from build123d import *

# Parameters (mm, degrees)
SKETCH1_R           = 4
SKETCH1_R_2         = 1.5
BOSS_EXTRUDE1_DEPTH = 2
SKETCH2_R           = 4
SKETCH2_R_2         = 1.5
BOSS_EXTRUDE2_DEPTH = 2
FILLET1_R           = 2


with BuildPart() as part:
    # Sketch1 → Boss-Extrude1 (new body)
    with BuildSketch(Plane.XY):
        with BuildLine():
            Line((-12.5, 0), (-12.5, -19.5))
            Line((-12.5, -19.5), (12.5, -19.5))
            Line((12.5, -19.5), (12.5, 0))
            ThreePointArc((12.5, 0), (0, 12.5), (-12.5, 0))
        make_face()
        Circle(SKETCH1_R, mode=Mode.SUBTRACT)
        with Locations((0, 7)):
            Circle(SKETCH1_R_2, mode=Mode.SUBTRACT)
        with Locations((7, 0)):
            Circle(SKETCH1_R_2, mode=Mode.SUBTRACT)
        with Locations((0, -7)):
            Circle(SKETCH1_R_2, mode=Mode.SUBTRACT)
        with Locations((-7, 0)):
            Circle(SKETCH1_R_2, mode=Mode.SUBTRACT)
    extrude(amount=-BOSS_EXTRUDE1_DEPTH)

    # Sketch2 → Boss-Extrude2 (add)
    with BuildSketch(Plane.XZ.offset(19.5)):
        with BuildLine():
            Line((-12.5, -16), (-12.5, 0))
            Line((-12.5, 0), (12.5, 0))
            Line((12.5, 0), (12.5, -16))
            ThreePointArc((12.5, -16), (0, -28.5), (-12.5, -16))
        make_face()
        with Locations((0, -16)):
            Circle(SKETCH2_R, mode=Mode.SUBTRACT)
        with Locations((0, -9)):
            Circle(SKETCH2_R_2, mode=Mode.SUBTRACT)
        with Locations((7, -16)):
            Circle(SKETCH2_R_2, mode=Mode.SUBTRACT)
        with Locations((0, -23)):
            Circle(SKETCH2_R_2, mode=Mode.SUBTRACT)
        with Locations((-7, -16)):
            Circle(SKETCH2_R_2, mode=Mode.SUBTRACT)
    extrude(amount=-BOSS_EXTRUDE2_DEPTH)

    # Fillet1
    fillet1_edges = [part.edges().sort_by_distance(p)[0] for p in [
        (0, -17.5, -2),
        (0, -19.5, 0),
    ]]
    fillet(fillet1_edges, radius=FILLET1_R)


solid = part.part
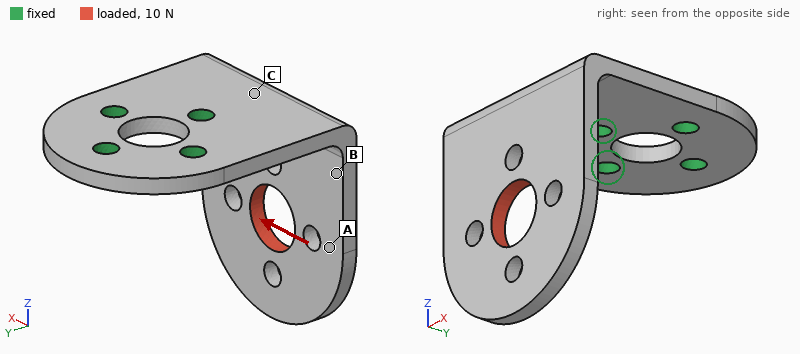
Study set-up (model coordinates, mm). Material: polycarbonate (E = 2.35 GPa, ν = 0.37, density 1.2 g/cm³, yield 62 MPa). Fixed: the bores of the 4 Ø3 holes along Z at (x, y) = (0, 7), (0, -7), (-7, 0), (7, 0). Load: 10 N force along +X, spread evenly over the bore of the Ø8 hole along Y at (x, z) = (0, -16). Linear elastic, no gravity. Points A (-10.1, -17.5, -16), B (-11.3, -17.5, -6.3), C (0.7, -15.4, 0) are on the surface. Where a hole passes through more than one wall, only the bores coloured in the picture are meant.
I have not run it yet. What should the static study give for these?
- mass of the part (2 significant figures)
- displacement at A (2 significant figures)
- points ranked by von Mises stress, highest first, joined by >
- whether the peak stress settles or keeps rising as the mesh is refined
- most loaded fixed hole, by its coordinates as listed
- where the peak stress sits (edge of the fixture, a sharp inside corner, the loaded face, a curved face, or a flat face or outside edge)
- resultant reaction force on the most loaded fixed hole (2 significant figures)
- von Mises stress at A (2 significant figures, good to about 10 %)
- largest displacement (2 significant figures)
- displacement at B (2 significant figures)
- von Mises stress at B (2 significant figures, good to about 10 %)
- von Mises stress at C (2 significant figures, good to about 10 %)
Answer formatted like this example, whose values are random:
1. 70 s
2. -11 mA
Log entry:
1. 2.8 g
2. 0.39 mm
3. C > B > A
4. keeps rising
5. (0, -7)
6. edge of the fixture
7. 11 N
8. 1.2 MPa
9. 0.58 mm
10. 0.26 mm
11. 2.9 MPa
12. 4.3 MPa
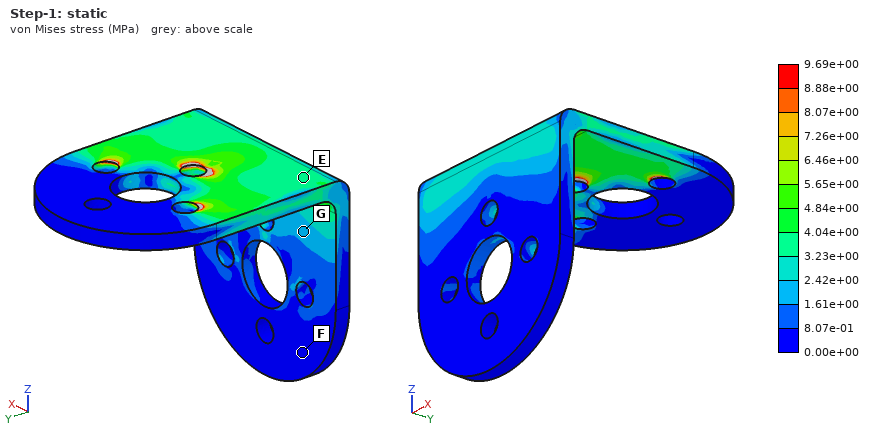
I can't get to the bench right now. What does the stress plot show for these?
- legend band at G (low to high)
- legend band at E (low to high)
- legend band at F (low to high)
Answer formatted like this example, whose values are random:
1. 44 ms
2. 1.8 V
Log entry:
1. 1.61e+00 to 2.42e+00 MPa
2. 3.23e+00 to 4.04e+00 MPa
3. 0.00e+00 to 8.07e-01 MPa
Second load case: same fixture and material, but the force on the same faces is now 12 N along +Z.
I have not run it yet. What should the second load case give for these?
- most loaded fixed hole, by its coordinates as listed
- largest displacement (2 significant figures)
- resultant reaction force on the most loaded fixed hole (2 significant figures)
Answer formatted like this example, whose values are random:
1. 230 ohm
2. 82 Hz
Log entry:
1. (0, -7)
2. 0.58 mm
3. 18 N
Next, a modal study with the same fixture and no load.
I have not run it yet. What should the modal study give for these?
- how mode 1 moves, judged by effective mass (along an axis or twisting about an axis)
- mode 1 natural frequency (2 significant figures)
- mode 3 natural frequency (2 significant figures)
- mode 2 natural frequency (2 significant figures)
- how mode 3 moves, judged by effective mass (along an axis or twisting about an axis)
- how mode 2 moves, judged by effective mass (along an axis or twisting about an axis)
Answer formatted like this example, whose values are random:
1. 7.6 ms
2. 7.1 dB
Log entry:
1. along Y
2. 470 Hz
3. 1500 Hz
4. 710 Hz
5. along Z
6. along X
